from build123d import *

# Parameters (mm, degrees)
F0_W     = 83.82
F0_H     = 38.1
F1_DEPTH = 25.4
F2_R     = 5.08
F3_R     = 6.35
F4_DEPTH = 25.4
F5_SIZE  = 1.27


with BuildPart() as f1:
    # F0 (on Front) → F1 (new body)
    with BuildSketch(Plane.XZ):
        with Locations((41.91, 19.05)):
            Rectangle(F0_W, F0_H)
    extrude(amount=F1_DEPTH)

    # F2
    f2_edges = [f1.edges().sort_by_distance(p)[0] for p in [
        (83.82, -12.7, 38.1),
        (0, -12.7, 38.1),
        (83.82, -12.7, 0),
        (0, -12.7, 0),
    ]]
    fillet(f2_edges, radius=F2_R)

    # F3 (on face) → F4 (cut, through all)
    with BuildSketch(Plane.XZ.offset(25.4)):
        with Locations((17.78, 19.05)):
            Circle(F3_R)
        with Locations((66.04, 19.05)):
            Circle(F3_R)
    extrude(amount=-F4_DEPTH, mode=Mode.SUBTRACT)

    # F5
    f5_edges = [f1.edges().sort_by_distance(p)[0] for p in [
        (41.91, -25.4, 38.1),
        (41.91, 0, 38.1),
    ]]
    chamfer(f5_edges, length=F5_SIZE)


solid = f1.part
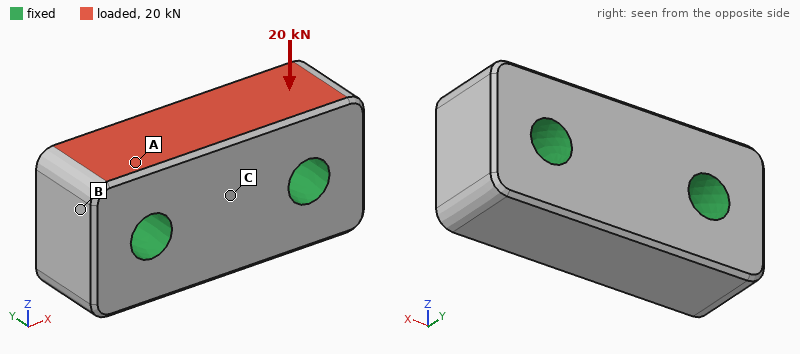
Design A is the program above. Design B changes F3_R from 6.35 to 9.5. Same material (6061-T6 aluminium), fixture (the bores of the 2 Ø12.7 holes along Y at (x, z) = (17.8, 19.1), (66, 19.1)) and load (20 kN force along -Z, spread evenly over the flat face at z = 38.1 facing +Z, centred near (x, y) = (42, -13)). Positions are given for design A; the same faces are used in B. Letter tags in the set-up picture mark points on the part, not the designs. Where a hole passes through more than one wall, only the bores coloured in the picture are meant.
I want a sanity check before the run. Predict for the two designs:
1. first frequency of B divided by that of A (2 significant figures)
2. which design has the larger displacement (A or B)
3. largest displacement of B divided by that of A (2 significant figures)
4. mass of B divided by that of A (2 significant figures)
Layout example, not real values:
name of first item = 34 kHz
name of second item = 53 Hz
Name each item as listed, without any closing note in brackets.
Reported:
first frequency of B divided by that of A = 1.3
which design has the larger displacement = A
largest displacement of B divided by that of A = 0.78
mass of B divided by that of A = 0.89
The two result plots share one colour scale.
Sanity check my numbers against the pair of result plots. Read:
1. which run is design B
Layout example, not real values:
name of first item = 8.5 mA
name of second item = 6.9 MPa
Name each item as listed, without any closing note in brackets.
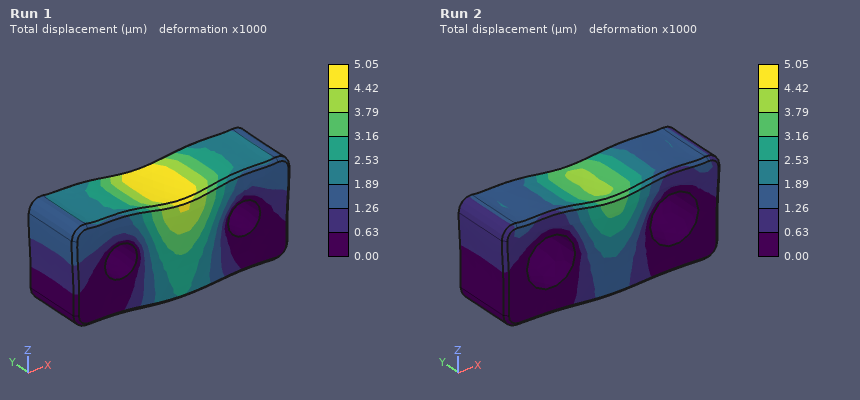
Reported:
which run is design B = Run 2
